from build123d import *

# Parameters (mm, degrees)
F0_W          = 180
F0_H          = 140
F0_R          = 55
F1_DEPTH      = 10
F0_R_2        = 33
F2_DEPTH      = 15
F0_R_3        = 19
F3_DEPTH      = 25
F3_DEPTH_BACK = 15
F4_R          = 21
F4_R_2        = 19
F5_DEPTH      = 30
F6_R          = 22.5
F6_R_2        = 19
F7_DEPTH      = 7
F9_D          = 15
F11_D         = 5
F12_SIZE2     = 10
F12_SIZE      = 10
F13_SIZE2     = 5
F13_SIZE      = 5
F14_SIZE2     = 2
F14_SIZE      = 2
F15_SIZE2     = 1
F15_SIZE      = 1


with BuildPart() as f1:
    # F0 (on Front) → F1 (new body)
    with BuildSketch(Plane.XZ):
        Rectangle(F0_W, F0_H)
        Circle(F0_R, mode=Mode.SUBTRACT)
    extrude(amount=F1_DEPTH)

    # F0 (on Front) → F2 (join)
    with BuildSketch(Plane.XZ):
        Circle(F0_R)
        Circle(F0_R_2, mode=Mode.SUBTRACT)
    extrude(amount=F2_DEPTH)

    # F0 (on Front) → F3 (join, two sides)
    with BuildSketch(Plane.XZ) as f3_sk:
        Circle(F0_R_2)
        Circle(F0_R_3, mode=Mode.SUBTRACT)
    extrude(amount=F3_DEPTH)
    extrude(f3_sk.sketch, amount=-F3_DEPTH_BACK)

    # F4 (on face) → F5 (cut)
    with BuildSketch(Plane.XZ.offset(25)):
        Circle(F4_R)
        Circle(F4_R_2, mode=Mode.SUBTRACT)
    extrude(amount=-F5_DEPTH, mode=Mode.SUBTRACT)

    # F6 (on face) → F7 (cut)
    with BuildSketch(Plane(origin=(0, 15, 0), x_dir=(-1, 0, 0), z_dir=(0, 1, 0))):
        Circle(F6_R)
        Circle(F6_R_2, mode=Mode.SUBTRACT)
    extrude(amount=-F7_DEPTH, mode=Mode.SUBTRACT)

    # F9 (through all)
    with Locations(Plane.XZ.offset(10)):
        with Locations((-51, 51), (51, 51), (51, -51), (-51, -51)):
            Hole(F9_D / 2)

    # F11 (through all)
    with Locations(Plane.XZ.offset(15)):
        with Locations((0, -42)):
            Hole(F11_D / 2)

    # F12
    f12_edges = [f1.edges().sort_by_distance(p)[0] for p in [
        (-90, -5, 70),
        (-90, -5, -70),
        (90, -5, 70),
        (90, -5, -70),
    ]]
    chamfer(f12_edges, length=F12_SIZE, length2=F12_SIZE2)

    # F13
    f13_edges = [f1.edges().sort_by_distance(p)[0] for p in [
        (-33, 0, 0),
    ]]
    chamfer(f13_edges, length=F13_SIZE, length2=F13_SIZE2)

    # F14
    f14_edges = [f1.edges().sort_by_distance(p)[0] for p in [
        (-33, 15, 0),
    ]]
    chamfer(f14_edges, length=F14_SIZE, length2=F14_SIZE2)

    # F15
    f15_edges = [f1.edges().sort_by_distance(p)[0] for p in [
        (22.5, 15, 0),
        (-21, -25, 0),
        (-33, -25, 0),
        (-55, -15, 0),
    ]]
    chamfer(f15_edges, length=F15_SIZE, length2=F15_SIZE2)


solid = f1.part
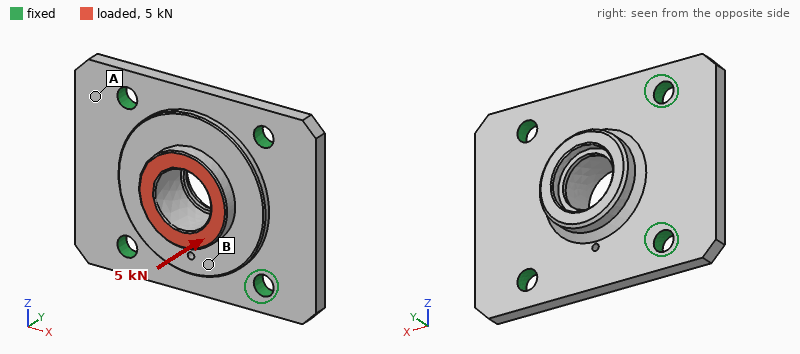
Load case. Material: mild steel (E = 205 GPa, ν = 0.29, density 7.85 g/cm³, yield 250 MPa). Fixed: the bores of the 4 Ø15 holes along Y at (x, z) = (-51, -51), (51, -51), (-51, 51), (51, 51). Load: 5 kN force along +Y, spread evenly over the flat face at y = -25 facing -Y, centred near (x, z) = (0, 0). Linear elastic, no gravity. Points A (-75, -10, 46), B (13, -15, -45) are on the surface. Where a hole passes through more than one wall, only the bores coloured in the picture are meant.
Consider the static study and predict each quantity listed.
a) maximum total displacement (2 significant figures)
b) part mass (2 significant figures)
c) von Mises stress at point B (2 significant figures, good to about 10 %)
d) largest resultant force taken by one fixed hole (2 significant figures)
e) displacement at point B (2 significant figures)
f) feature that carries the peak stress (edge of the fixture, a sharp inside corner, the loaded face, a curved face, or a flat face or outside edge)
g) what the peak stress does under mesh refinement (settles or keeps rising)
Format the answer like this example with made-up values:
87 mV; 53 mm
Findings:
5.3 µm; 2.5 kg; 5.9 MPa; 1.4 kN; 3.7 µm; edge of the fixture; keeps rising
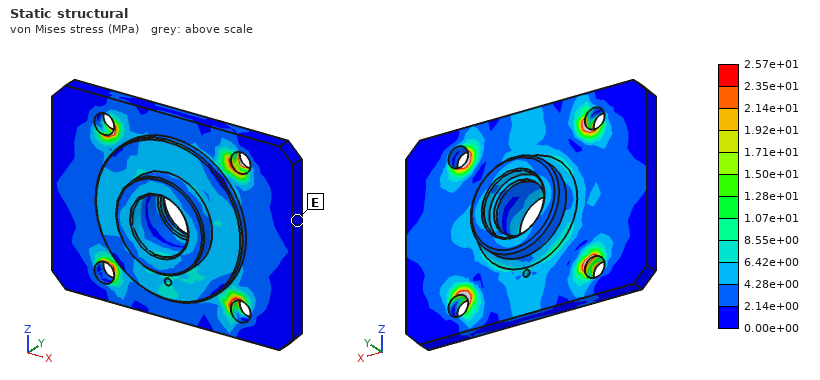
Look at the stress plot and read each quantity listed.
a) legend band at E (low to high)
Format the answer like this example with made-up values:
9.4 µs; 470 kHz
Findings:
0.00e+00 to 2.14e+00 MPa
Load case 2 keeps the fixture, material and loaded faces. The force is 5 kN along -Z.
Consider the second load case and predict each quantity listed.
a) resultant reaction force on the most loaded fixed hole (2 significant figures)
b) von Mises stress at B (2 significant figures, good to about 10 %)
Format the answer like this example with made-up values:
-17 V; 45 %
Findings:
1.5 kN; 2.8 MPa
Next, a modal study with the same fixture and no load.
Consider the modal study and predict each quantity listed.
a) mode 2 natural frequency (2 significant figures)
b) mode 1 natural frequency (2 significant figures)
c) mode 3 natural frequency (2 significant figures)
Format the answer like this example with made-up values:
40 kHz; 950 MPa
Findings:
4500 Hz; 4400 Hz; 4900 Hz
